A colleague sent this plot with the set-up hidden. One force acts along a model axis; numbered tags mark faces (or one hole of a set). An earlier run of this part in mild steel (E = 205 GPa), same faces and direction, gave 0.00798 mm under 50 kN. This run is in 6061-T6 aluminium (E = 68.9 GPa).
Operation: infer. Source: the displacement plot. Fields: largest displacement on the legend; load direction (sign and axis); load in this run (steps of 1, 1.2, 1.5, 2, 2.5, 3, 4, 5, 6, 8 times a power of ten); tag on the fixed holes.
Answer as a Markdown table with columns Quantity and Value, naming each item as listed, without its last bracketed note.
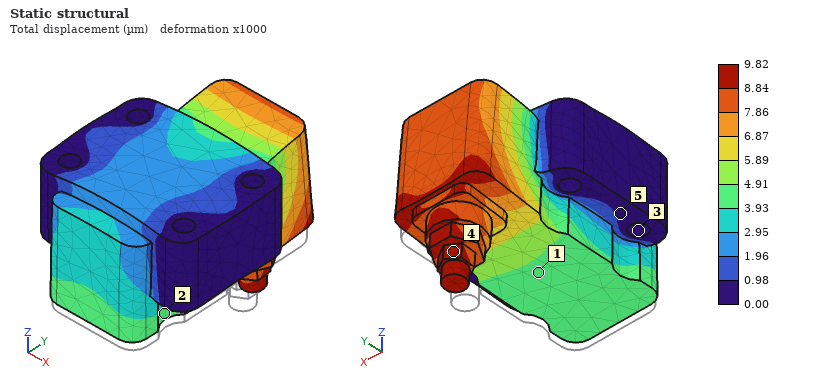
| Quantity | Value |
|---|---|
| largest displacement on the legend | 9.82 µm |
| load direction | +Z |
| load in this run | 20 kN |
| tag on the fixed holes | 3 |
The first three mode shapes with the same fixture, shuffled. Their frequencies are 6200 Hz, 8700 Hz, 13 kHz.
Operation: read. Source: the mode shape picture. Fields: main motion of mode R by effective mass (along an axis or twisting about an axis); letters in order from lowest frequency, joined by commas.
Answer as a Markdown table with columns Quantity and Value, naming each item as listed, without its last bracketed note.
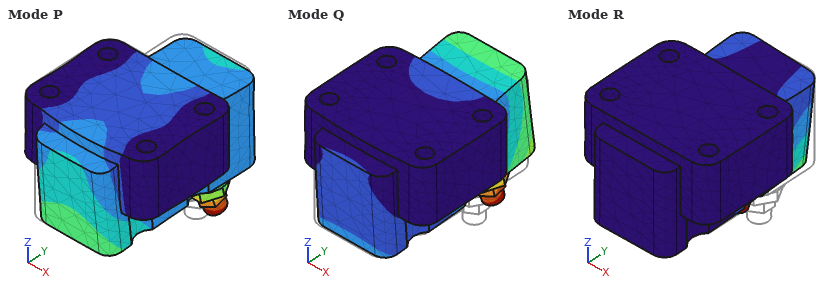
| Quantity | Value |
|---|---|
| main motion of mode R by effective mass | along X |
| letters in order from lowest frequency, joined by commas | Q, R, P |
